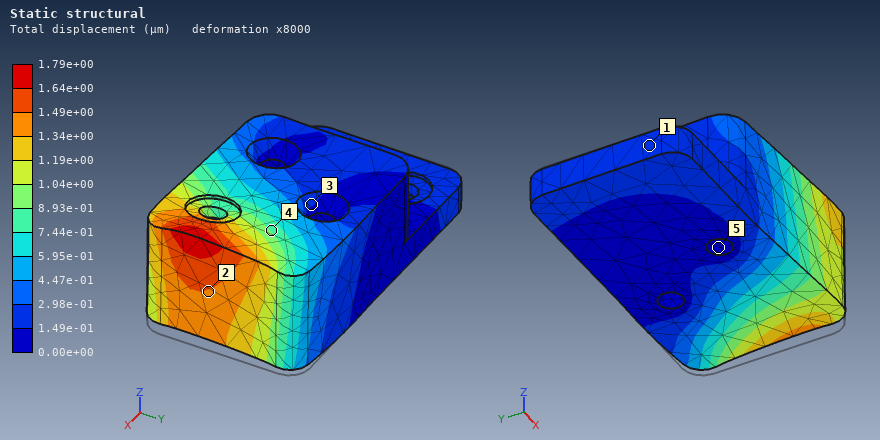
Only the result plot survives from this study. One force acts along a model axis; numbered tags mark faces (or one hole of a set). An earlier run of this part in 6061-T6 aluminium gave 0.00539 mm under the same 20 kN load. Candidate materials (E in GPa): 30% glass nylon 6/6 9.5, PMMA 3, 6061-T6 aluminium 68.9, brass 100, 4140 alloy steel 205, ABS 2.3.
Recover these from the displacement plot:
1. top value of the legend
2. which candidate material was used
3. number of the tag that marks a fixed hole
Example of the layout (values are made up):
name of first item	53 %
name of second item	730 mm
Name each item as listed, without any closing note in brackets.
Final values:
top value of the legend	1.79e+00 µm
which candidate material was used	4140 alloy steel
number of the tag that marks a fixed hole	5
